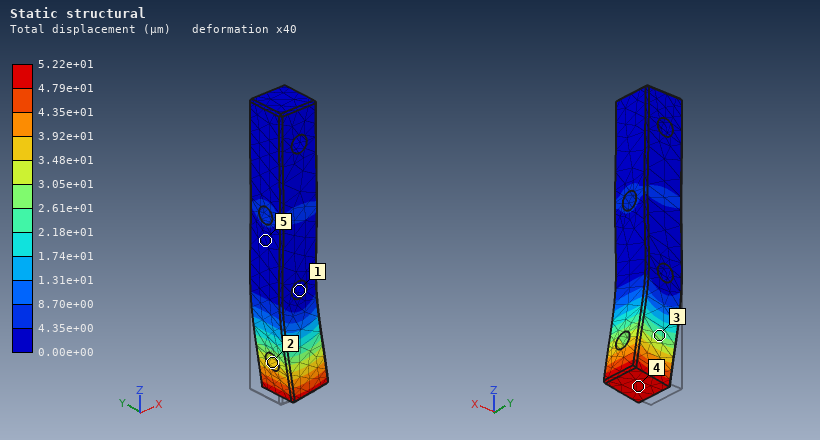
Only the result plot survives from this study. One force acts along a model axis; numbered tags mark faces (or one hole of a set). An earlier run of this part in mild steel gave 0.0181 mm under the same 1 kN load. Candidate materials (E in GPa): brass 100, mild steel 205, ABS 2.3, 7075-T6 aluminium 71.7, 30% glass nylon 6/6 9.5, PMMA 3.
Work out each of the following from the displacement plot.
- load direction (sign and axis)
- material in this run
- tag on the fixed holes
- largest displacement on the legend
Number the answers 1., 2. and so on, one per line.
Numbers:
1. +X
2. 7075-T6 aluminium
3. 1
4. 5.22e+01 µm
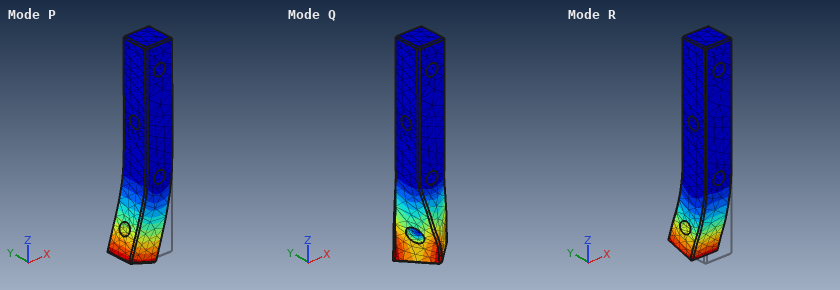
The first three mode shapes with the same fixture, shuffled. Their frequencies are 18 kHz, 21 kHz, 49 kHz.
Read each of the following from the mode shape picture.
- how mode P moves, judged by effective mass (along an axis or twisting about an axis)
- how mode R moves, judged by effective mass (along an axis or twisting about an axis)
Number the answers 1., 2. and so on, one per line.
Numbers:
1. along X
2. along Y
